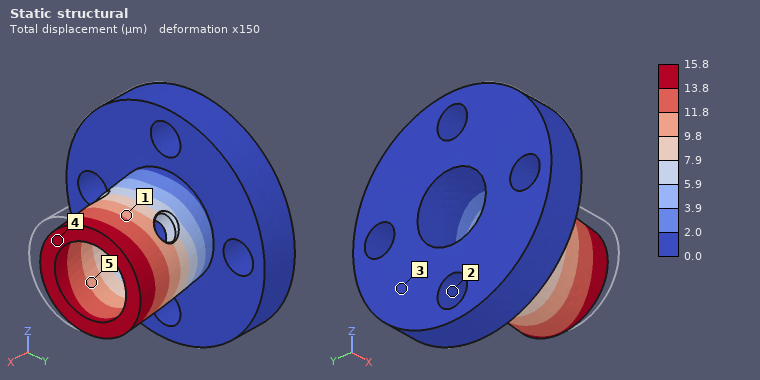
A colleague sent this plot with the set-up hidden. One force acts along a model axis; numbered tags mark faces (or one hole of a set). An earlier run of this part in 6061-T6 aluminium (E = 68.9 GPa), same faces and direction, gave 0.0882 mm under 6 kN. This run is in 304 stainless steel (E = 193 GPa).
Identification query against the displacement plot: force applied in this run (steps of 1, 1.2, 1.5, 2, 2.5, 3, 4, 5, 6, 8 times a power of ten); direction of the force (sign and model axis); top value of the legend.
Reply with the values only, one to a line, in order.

3 kN
+Y
15.8 µm
